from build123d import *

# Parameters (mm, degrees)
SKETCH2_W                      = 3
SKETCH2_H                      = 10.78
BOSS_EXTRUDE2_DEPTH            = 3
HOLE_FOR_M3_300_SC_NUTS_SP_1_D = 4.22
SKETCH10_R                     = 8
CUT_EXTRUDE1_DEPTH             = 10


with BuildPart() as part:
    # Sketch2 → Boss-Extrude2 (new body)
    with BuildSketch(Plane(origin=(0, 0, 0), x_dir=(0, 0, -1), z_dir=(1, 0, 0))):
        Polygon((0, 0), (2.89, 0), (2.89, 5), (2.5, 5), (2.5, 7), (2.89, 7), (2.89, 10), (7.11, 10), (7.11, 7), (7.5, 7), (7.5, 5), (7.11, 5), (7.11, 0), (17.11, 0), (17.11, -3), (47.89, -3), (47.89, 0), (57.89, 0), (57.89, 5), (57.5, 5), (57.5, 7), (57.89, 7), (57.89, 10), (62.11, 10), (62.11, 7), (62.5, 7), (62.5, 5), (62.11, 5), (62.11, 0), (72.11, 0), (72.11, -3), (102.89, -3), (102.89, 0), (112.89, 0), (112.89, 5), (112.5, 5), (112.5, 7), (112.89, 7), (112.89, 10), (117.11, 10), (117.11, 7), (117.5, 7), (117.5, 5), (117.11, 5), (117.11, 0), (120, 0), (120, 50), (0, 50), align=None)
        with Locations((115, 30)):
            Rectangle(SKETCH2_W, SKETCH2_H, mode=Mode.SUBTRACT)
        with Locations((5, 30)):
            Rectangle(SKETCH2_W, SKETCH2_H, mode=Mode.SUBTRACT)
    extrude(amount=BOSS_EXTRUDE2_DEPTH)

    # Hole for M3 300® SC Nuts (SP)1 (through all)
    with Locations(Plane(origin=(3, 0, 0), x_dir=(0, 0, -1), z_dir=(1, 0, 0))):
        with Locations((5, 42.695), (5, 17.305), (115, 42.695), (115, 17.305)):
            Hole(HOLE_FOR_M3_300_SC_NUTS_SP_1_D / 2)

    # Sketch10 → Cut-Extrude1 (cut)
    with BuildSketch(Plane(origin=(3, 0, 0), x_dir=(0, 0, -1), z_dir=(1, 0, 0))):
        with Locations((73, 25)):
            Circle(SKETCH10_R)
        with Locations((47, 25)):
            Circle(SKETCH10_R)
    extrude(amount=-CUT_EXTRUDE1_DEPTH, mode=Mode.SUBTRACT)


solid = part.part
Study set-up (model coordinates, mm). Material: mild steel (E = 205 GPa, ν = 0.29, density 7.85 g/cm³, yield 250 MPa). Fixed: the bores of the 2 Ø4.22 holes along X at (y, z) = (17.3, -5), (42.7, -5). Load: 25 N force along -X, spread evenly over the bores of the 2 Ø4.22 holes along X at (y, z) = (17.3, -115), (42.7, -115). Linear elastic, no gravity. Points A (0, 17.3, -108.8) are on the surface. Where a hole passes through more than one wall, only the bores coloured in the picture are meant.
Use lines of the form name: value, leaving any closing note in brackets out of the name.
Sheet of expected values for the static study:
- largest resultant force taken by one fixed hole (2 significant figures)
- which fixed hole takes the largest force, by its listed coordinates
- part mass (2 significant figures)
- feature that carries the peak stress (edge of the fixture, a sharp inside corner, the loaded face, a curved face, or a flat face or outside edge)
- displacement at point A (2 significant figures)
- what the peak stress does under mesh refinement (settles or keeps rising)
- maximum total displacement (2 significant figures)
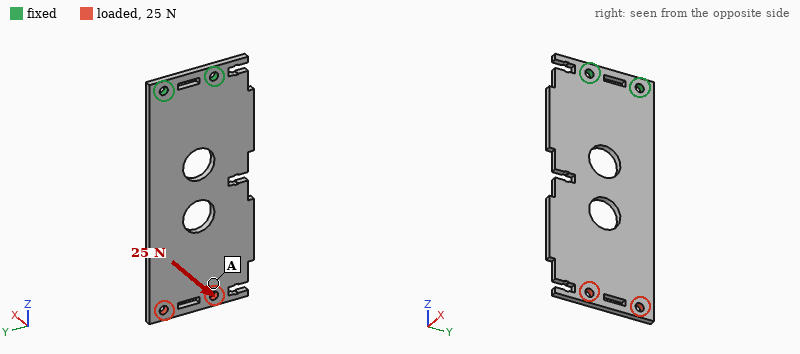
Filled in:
largest resultant force taken by one fixed hole: 18 N
which fixed hole takes the largest force, by its listed coordinates: (17.3, -5)
part mass: 130 g
feature that carries the peak stress: edge of the fixture
displacement at point A: 0.52 mm
what the peak stress does under mesh refinement: keeps rising
maximum total displacement: 0.62 mm
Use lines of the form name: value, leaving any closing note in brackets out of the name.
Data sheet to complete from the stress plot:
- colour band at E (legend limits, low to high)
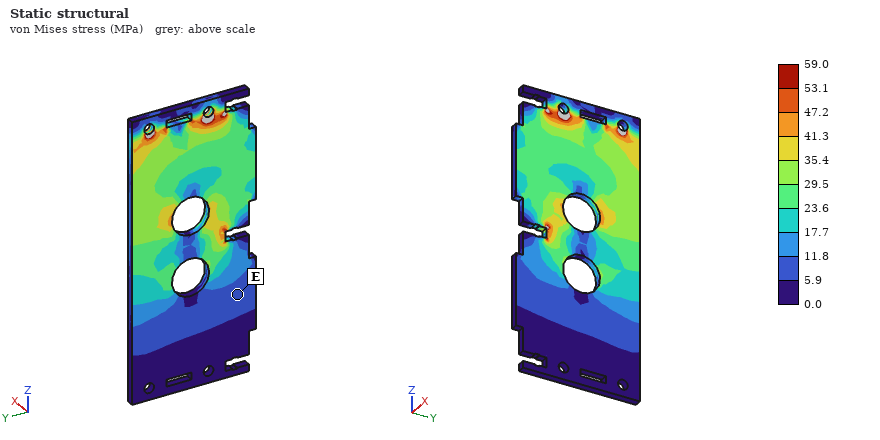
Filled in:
colour band at E: 5.9 to 11.8 MPa
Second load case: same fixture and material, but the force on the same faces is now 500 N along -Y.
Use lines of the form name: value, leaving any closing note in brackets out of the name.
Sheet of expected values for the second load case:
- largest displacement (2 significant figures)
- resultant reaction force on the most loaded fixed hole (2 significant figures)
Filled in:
largest displacement: 77 µm
resultant reaction force on the most loaded fixed hole: 2.0 kN
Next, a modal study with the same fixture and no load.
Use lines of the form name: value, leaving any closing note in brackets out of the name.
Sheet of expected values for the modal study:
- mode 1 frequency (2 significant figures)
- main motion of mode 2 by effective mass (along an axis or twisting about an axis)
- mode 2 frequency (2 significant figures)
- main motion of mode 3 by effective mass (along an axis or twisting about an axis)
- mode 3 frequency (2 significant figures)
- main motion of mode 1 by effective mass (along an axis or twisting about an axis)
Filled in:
mode 1 frequency: 180 Hz
main motion of mode 2 by effective mass: twisting about Z
mode 2 frequency: 790 Hz
main motion of mode 3 by effective mass: along X
mode 3 frequency: 1100 Hz
main motion of mode 1 by effective mass: along X
